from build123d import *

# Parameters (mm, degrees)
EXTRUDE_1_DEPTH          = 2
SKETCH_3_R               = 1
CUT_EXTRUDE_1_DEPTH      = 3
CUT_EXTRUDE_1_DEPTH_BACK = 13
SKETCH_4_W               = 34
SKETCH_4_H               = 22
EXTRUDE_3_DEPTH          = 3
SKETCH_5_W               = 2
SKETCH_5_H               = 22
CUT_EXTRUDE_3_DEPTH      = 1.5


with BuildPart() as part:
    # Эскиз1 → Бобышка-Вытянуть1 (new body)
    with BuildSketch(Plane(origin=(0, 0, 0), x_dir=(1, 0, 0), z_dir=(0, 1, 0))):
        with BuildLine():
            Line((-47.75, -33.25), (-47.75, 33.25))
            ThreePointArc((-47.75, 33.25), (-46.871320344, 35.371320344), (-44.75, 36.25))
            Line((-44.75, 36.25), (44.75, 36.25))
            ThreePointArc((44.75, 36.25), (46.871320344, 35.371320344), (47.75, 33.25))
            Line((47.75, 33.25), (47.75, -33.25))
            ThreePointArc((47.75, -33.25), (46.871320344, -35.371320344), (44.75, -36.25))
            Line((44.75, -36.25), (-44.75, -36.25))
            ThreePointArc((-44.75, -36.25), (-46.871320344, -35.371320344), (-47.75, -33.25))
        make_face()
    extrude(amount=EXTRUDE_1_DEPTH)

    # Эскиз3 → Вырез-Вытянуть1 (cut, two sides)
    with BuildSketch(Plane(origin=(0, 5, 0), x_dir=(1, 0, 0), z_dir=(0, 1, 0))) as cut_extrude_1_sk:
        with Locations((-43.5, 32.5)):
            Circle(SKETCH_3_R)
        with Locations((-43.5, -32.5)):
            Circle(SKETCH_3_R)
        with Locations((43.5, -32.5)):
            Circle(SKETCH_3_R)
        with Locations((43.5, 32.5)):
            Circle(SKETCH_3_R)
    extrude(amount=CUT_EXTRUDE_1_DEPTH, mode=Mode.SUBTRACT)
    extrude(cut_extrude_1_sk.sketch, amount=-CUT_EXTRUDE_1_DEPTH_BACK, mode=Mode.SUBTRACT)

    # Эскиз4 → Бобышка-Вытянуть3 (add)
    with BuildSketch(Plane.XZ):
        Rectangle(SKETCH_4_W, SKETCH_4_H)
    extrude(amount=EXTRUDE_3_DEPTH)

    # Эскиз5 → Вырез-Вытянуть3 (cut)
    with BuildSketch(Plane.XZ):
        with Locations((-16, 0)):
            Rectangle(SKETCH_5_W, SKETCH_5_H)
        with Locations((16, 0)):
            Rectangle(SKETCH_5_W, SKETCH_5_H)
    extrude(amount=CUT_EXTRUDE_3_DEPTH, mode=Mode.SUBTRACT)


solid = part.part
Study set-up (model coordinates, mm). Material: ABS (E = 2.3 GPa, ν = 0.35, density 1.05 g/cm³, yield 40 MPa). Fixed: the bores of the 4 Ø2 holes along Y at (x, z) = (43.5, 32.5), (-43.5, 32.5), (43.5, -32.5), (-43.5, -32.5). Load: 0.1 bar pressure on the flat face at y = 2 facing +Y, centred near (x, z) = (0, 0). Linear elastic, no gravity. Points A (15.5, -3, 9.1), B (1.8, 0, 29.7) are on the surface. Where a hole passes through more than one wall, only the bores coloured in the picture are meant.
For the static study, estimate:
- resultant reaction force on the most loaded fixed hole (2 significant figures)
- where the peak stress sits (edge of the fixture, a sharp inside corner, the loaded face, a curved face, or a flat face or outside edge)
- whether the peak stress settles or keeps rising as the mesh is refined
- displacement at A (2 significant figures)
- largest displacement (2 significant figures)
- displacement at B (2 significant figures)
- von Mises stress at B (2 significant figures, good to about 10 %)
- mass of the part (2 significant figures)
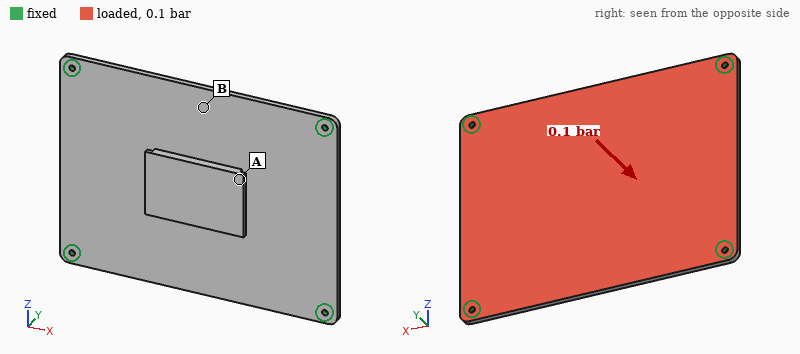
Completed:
18 N
edge of the fixture
keeps rising
1.3 mm
1.4 mm
1.3 mm
4.5 MPa
17 g
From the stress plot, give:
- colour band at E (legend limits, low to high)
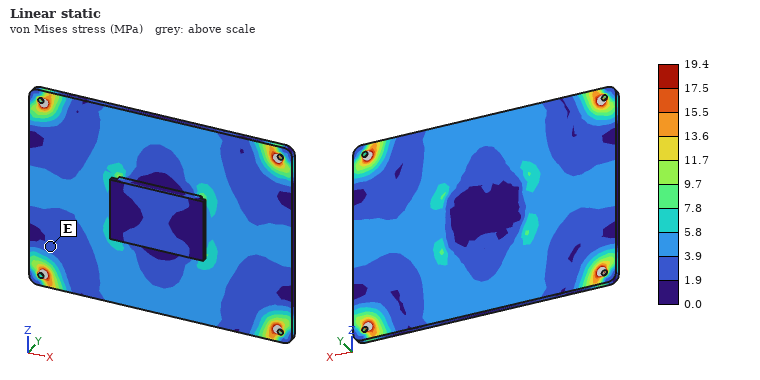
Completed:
1.9 to 3.9 MPa
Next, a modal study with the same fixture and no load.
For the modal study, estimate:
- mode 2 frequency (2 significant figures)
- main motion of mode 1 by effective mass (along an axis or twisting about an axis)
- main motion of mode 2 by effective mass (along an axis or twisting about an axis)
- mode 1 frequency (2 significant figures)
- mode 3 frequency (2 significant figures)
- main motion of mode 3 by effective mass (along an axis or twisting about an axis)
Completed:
500 Hz
along Y
twisting about X
290 Hz
650 Hz
twisting about Z
